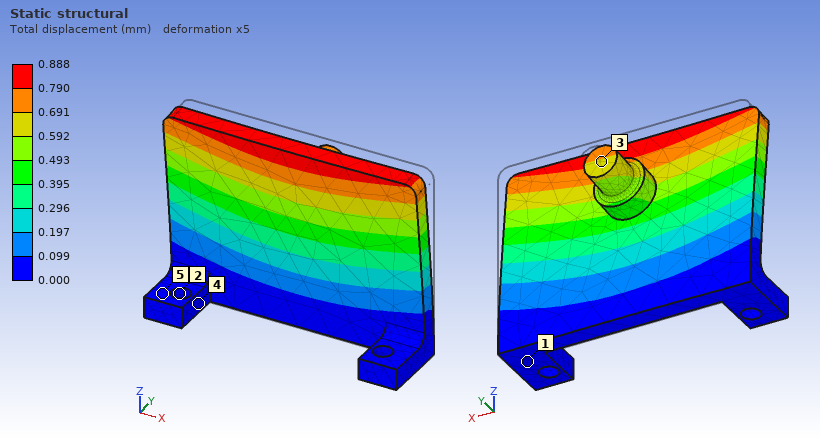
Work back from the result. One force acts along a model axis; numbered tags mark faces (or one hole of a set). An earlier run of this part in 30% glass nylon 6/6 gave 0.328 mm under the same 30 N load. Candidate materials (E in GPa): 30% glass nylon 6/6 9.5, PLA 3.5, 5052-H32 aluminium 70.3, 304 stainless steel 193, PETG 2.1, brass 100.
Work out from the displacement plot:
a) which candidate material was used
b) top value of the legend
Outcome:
PLA
0.888 mm
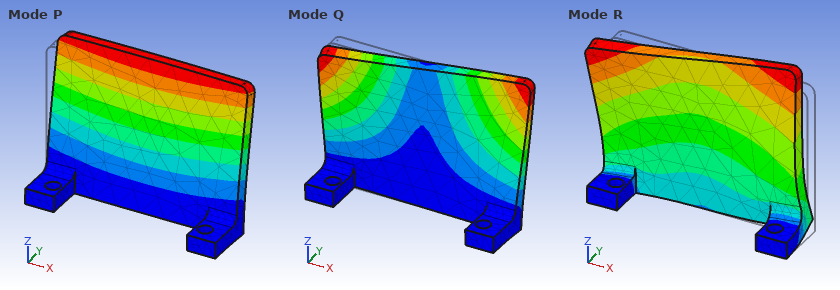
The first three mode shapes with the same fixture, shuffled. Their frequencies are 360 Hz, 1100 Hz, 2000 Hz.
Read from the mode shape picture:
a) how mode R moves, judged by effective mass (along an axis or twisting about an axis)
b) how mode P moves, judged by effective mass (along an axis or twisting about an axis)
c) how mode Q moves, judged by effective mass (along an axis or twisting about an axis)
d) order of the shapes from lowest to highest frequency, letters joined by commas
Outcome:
along X
along Y
twisting about Z
P, Q, R
